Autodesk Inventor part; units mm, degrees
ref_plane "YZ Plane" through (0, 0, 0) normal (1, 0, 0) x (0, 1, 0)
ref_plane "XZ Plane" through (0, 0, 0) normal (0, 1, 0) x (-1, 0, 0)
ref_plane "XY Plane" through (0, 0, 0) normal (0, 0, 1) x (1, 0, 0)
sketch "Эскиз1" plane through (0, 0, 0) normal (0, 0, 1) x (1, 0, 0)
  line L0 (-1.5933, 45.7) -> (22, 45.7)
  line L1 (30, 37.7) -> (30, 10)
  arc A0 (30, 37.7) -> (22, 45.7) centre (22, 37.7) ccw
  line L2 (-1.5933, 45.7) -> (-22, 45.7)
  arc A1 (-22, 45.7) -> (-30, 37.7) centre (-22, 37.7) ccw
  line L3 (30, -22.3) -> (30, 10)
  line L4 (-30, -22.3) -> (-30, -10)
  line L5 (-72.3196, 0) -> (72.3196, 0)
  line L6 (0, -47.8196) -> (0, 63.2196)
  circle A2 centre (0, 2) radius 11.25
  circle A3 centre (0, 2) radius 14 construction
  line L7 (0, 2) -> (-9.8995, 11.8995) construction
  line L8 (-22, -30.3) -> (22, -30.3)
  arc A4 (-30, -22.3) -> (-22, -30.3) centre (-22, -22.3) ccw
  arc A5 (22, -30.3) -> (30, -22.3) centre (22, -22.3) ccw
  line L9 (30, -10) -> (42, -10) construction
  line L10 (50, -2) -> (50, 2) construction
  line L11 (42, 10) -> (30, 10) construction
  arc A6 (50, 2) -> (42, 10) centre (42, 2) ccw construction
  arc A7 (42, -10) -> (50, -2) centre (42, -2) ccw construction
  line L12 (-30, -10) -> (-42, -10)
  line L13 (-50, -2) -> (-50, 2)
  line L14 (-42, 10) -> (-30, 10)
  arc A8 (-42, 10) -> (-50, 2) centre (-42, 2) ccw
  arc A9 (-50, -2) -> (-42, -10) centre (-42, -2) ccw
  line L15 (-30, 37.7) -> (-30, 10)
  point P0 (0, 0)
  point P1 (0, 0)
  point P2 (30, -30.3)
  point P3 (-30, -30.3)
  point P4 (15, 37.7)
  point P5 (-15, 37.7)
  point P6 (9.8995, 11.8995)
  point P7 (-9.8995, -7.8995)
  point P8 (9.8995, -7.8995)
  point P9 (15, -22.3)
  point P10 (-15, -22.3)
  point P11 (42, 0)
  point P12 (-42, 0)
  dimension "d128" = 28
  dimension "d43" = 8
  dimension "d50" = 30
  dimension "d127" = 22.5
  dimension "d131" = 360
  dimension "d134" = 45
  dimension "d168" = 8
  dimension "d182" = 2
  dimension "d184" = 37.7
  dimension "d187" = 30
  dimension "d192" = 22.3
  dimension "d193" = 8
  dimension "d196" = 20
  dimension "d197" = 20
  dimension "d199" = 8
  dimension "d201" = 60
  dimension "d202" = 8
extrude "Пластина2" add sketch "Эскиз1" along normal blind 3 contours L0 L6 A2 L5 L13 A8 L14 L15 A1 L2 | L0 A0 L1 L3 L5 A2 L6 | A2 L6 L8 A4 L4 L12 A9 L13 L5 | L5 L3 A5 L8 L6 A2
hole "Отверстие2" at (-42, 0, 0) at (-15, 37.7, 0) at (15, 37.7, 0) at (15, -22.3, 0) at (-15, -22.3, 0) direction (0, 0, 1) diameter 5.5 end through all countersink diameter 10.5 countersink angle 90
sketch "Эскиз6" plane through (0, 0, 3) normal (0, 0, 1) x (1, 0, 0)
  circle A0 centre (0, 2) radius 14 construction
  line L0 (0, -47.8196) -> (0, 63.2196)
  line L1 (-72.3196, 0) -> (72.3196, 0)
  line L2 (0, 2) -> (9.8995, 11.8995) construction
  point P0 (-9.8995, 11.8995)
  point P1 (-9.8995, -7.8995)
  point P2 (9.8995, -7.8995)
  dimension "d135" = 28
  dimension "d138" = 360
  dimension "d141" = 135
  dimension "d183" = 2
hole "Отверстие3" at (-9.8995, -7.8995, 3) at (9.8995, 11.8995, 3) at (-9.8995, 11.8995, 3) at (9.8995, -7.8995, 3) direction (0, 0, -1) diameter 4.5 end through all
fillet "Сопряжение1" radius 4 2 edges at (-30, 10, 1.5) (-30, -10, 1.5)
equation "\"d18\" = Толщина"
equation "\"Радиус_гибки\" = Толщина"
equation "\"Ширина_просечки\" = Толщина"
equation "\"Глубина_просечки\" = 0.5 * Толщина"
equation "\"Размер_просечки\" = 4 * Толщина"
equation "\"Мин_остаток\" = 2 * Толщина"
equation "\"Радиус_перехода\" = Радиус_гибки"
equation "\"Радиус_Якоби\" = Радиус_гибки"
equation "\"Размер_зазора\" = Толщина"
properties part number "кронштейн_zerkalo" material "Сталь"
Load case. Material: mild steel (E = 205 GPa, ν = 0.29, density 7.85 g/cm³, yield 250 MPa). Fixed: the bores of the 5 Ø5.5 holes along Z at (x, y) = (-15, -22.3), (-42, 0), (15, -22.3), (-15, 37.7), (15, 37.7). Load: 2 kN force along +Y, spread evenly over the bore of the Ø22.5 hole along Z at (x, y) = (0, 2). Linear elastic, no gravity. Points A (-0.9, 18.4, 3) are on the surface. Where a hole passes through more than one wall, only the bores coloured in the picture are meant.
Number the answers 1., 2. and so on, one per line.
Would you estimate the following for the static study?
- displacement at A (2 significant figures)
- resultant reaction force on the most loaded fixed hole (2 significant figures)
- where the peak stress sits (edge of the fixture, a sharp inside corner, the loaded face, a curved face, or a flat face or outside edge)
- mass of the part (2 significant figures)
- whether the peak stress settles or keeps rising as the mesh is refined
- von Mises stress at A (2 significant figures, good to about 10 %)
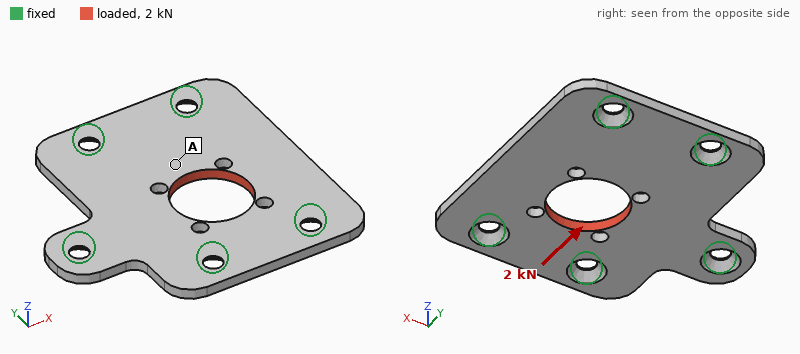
1. 1.9 µm
2. 540 N
3. edge of the fixture
4. 99 g
5. keeps rising
6. 12 MPa
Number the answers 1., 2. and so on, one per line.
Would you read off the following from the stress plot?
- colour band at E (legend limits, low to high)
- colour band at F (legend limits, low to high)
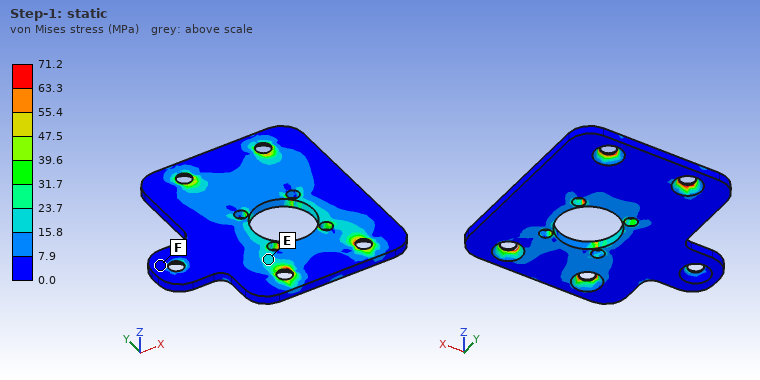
1. 15.8 to 23.7 MPa
2. 0.0 to 7.9 MPa
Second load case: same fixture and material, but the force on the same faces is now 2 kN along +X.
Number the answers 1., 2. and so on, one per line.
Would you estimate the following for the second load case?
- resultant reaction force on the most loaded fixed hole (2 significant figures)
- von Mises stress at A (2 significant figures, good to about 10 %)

1. 450 N
2. 12 MPa
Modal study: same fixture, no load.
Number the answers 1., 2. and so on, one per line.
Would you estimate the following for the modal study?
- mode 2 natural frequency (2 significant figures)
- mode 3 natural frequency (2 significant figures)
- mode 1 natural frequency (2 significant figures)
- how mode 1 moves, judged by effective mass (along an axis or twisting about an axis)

1. 4900 Hz
2. 7500 Hz
3. 3400 Hz
4. along Z
